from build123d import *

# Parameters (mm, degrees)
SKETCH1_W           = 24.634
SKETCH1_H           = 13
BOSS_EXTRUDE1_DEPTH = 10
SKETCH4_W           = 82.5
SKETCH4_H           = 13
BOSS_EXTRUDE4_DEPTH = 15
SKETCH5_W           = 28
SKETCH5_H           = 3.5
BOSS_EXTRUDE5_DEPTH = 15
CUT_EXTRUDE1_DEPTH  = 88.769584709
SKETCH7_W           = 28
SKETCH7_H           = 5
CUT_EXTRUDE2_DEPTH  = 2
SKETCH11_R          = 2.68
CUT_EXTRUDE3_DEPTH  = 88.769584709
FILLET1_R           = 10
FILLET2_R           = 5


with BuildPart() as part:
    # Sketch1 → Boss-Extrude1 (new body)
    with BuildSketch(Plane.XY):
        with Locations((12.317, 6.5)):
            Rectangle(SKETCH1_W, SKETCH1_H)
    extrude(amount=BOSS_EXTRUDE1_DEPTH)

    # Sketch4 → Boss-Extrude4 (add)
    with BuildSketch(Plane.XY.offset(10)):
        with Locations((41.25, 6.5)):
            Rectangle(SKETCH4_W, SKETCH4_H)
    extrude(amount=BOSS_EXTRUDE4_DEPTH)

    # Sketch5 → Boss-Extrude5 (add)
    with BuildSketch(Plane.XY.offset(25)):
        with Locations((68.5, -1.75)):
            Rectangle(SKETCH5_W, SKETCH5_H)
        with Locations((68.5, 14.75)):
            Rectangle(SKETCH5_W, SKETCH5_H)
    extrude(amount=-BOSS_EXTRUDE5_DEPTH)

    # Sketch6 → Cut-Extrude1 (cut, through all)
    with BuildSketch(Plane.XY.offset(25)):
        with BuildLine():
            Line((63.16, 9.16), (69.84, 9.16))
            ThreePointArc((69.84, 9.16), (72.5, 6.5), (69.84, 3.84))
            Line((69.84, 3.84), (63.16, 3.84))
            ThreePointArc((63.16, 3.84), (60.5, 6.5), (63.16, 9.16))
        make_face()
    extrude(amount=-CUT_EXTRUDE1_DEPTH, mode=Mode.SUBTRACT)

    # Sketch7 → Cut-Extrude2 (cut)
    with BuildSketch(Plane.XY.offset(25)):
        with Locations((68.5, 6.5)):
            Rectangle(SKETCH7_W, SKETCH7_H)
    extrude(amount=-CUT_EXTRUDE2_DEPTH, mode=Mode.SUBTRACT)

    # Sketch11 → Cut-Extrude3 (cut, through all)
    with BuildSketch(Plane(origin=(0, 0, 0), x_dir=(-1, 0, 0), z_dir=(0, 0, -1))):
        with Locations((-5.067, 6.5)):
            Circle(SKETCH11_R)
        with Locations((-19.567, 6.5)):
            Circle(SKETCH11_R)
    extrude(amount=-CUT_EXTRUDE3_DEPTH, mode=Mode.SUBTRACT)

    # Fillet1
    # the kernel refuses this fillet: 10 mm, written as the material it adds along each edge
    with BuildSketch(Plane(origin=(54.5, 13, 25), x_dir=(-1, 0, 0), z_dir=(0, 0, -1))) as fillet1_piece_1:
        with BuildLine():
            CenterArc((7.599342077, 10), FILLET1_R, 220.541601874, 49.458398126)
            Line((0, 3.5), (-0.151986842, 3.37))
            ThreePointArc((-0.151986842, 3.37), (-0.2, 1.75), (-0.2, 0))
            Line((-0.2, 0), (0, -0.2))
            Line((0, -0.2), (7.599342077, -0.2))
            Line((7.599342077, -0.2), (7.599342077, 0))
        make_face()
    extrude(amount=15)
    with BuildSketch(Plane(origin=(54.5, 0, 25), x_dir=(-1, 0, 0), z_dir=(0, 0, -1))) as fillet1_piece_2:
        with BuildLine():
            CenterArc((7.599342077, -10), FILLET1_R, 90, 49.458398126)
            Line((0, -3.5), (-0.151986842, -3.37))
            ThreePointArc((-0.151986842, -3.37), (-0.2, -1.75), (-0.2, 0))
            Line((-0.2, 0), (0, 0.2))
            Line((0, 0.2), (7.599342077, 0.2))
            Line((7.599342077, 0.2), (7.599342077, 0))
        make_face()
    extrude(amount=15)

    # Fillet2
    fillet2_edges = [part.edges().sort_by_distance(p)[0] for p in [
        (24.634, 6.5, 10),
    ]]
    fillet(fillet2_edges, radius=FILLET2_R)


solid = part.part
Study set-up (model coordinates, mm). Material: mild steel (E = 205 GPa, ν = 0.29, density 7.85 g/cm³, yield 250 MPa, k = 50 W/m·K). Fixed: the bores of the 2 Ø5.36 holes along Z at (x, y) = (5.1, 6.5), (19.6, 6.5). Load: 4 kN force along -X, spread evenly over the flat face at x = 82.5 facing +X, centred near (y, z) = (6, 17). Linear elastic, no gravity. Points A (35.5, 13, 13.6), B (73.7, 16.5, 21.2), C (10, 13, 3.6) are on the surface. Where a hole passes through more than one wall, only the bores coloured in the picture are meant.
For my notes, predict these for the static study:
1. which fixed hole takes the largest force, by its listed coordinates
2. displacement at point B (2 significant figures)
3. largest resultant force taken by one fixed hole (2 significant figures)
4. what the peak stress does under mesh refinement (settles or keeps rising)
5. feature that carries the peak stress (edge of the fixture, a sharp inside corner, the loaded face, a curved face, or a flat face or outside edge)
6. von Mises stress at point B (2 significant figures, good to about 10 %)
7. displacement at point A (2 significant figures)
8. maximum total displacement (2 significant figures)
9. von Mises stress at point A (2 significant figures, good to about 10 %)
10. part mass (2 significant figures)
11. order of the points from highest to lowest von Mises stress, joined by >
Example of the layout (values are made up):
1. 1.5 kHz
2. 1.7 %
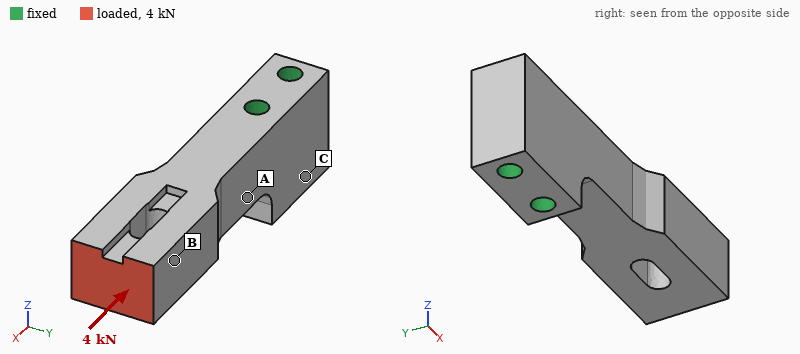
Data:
1. (19.6, 6.5)
2. 4.8 µm
3. 3.7 kN
4. keeps rising
5. edge of the fixture
6. 16 MPa
7. 1.4 µm
8. 6.0 µm
9. 21 MPa
10. 160 g
11. A > B > C
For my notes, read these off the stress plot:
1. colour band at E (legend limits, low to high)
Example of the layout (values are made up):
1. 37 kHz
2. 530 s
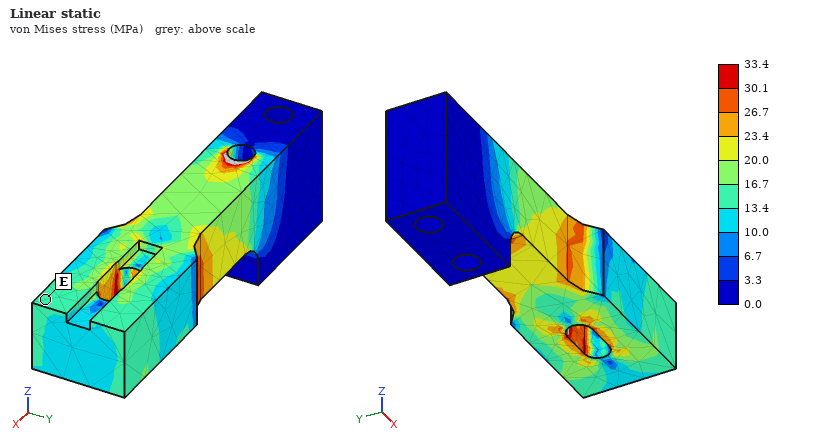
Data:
1. 13.4 to 16.7 MPa
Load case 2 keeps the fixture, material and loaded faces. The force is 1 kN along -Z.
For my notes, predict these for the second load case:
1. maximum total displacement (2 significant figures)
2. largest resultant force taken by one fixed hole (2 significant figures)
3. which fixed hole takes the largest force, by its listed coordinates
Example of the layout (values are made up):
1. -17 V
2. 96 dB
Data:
1. 100 µm
2. 1.1 kN
3. (19.6, 6.5)
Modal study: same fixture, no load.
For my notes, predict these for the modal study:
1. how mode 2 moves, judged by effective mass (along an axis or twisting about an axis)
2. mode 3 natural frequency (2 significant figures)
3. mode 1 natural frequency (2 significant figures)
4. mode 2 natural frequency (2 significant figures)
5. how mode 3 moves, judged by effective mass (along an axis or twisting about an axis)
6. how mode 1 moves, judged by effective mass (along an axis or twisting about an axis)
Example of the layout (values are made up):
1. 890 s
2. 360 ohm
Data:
1. along Z
2. 8800 Hz
3. 2200 Hz
4. 2800 Hz
5. twisting about X
6. along Y
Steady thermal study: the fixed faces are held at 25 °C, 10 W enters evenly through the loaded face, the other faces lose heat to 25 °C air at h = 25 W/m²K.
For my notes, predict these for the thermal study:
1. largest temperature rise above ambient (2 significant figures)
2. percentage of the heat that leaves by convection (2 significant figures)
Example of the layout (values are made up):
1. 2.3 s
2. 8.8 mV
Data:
1. 45 K
2. 27 %
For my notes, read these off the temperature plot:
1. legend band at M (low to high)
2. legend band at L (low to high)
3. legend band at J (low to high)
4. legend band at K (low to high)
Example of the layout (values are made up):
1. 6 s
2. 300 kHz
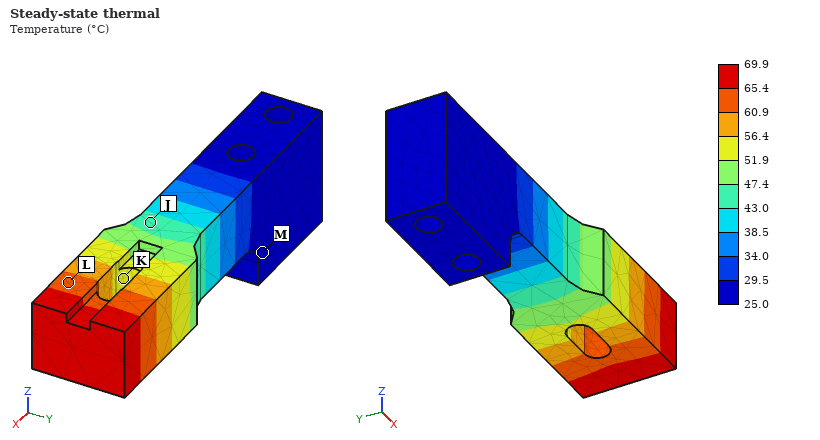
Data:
1. 25.0 to 29.5 °C
2. 60.9 to 65.4 °C
3. 43.0 to 47.4 °C
4. 51.9 to 56.4 °C
